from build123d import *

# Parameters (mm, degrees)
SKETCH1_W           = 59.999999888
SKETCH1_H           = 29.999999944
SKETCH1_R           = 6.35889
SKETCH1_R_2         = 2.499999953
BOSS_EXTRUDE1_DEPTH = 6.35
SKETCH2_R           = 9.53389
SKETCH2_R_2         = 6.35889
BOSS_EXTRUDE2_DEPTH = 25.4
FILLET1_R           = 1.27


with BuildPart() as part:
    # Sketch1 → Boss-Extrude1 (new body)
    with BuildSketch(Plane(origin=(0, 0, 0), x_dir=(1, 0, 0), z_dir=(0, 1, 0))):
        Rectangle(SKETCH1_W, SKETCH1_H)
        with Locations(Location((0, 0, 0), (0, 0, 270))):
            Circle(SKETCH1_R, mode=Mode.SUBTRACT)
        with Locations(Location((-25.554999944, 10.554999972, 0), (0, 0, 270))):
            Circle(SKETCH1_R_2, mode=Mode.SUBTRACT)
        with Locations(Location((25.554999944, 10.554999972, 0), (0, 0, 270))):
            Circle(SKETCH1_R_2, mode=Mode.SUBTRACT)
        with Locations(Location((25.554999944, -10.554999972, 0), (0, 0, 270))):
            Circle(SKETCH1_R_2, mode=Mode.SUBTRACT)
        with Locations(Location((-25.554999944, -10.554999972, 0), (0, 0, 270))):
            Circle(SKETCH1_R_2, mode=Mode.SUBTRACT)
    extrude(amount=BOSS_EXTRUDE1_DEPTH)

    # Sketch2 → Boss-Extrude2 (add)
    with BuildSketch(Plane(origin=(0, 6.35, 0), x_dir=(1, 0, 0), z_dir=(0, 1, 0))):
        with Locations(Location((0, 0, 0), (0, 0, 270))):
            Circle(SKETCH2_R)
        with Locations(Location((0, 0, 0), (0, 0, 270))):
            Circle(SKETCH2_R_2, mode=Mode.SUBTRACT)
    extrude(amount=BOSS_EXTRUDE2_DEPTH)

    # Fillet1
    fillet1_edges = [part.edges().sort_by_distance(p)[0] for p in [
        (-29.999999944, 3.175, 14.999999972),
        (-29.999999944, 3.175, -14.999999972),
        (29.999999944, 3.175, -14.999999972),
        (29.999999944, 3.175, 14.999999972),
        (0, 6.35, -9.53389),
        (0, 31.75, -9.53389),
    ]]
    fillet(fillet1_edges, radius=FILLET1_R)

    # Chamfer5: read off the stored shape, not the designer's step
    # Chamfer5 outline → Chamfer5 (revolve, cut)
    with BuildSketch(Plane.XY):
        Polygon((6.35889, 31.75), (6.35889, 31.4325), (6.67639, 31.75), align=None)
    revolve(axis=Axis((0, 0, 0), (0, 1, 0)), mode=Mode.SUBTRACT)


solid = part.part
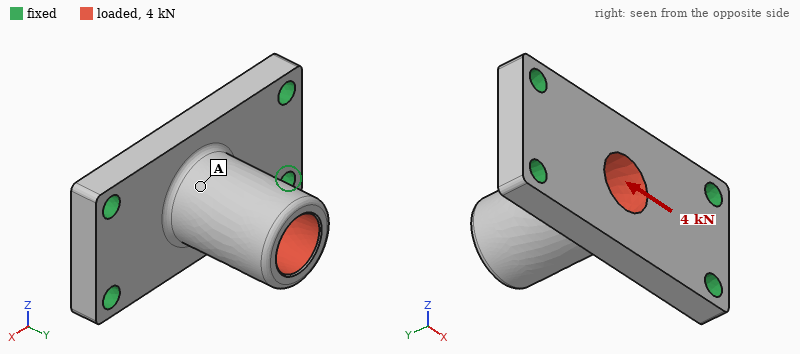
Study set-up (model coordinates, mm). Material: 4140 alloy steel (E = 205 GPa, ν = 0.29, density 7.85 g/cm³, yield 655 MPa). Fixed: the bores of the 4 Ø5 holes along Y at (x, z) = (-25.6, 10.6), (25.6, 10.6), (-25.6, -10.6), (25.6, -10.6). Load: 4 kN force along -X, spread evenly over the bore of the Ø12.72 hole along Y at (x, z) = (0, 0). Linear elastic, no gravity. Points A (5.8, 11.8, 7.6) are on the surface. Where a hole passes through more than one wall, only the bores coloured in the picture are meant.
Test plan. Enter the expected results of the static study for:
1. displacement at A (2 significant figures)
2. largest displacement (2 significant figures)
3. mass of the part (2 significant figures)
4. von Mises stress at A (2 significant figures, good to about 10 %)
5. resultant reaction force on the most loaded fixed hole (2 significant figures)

10 µm
33 µm
110 g
32 MPa
1.2 kN
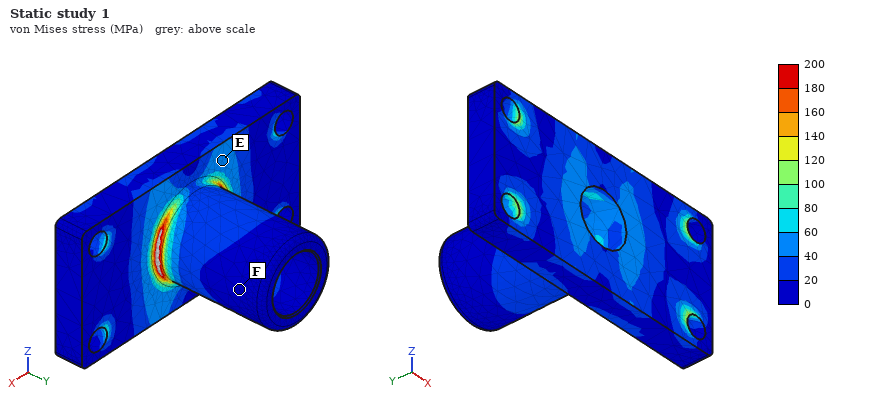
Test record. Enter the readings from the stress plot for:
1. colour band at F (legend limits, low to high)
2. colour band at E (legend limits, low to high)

0 to 20 MPa
40 to 60 MPa
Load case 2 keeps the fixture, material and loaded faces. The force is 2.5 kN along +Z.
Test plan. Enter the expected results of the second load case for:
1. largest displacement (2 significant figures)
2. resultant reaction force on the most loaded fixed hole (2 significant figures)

39 µm
1.2 kN
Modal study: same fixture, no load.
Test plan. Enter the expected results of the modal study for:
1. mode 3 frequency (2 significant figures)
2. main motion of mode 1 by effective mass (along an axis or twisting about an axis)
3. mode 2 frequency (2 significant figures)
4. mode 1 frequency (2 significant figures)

10 kHz
along Z
9900 Hz
7200 Hz
